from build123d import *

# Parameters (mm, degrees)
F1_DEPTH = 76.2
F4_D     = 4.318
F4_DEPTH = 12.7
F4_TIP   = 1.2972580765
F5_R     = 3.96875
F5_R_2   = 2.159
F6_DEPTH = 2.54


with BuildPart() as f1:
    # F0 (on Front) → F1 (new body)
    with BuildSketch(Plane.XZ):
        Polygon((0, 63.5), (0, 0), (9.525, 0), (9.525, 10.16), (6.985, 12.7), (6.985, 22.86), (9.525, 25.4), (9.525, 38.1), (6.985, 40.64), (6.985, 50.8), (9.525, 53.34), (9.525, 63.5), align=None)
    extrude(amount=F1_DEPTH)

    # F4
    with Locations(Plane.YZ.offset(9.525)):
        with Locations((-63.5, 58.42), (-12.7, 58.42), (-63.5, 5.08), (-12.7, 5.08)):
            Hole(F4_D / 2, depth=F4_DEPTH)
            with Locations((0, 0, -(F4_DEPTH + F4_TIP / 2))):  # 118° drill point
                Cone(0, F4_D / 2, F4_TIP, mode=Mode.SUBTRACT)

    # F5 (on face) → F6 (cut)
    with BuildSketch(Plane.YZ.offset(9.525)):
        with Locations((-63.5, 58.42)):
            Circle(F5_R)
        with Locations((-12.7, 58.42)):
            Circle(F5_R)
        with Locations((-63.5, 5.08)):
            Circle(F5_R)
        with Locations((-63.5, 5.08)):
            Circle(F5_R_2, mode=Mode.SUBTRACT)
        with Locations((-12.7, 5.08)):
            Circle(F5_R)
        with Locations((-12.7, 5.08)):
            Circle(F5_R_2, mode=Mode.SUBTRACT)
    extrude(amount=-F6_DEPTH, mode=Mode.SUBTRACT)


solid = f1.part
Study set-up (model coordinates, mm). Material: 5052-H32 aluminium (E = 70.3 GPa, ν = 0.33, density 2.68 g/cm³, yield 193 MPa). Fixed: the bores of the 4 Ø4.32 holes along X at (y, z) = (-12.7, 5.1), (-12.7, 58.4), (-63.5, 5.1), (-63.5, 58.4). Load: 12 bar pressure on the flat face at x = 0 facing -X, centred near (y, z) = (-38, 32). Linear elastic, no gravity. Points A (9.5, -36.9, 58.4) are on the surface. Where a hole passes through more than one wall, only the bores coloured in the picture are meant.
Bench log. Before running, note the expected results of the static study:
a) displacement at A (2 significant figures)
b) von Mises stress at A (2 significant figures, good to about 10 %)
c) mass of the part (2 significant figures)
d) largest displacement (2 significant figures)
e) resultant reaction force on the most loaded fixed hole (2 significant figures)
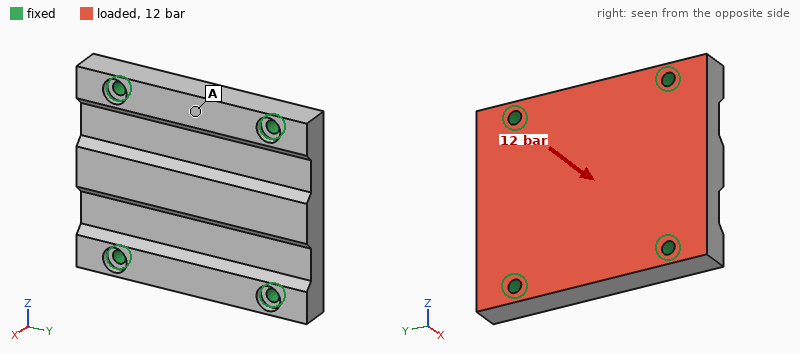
12 µm
17 MPa
110 g
23 µm
1.4 kN
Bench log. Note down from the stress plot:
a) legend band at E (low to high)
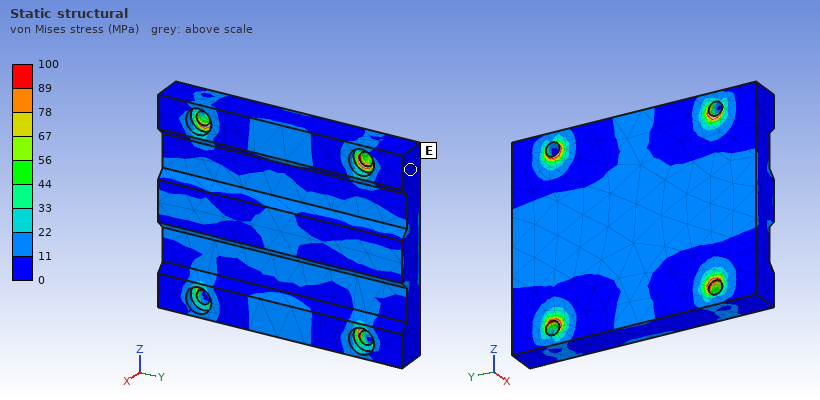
0 to 11 MPa
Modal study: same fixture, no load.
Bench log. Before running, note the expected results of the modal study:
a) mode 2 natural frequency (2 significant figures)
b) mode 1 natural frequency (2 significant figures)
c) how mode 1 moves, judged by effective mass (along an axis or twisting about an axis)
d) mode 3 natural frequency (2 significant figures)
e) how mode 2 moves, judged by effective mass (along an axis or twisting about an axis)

12 kHz
8900 Hz
along X
13 kHz
twisting about Z
